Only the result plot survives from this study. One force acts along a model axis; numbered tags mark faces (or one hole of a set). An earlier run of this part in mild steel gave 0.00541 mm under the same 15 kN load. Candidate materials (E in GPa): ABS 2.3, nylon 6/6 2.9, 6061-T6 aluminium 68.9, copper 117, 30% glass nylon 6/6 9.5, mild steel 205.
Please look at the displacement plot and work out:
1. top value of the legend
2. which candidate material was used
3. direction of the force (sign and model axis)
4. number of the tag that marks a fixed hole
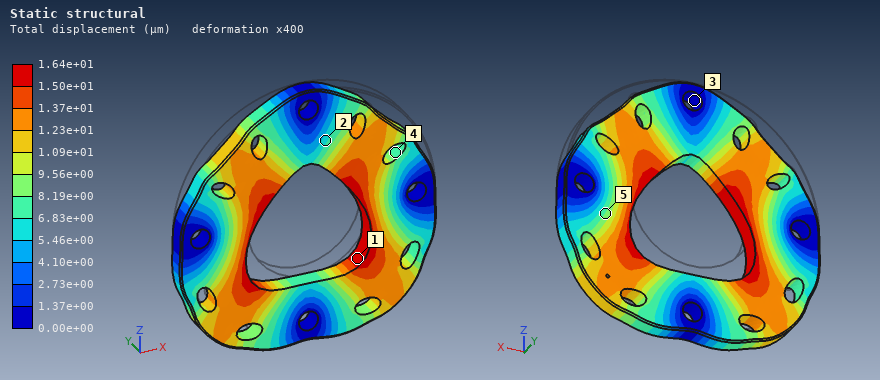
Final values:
1.64e+01 µm
6061-T6 aluminium
-Z
3
